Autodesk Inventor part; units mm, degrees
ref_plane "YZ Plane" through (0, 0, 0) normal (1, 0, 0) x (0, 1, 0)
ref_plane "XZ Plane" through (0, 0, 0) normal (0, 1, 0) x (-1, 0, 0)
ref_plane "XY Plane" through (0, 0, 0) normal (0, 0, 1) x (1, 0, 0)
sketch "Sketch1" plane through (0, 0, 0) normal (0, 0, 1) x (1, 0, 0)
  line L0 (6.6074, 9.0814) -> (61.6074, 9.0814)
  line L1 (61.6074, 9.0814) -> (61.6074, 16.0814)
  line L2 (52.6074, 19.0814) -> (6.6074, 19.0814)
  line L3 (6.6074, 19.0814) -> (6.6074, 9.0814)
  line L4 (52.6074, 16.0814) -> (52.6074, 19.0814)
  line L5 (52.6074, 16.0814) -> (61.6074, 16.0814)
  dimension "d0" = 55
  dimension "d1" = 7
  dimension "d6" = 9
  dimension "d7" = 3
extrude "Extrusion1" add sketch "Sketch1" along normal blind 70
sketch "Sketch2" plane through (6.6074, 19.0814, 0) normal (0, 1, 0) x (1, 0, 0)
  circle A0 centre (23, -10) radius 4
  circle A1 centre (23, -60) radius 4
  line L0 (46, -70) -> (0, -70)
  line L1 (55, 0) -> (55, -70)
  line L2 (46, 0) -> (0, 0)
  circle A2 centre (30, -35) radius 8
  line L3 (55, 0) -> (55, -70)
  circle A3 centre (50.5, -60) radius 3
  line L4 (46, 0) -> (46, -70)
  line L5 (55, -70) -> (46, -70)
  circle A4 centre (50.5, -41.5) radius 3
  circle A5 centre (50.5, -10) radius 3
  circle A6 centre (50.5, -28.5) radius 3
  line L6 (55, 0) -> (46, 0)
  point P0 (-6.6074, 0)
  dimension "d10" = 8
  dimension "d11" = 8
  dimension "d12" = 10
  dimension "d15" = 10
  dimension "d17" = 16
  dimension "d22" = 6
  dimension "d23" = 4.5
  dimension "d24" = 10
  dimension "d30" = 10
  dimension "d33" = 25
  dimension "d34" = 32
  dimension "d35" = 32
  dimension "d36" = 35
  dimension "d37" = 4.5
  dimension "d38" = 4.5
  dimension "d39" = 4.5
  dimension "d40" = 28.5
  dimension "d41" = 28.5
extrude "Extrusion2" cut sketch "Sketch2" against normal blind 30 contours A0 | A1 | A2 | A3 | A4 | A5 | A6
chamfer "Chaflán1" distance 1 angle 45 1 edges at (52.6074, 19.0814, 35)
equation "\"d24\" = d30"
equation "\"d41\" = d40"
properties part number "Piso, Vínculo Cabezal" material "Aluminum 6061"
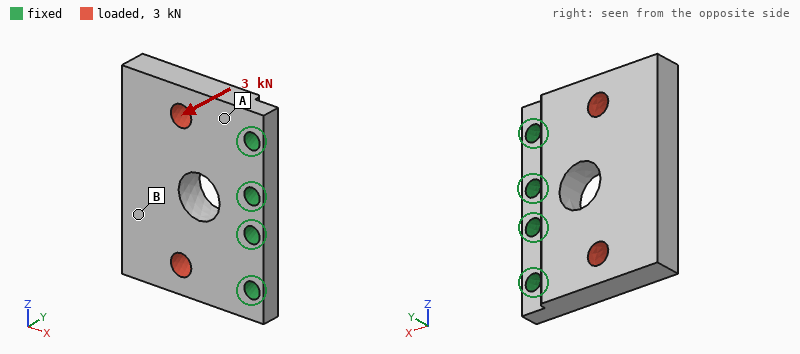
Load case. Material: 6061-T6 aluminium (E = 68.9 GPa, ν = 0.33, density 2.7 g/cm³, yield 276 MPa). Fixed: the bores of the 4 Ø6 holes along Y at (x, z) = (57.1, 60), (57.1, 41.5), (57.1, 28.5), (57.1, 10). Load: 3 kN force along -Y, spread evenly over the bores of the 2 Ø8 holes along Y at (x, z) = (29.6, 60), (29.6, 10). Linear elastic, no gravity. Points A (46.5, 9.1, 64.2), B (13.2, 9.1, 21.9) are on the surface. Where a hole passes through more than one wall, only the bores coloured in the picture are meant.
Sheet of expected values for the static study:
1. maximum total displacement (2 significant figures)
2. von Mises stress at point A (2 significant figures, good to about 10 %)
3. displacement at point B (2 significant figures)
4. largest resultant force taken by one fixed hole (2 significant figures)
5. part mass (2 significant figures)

0.22 mm
51 MPa
0.18 mm
980 N
88 g
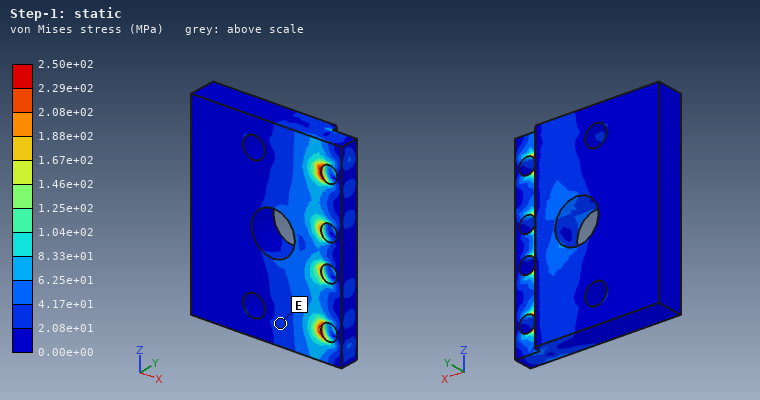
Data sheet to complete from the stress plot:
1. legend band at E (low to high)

2.08e+01 to 4.17e+01 MPa
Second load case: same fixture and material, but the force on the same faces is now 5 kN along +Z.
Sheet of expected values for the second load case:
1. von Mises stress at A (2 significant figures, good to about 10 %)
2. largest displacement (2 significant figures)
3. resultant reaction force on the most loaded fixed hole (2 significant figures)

15 MPa
24 µm
2.7 kN
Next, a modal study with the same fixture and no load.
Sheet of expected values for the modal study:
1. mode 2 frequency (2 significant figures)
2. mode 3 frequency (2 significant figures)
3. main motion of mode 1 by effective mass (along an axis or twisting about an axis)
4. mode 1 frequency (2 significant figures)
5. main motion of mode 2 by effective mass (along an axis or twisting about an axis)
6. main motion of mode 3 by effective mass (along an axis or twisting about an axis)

4800 Hz
9400 Hz
along Y
2400 Hz
twisting about X
along Z
